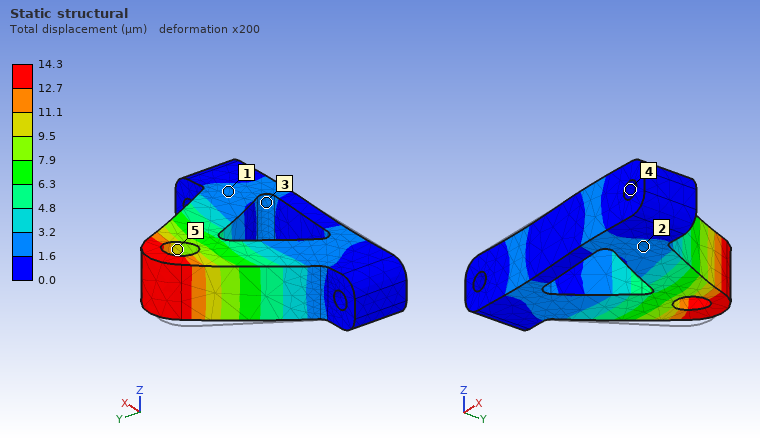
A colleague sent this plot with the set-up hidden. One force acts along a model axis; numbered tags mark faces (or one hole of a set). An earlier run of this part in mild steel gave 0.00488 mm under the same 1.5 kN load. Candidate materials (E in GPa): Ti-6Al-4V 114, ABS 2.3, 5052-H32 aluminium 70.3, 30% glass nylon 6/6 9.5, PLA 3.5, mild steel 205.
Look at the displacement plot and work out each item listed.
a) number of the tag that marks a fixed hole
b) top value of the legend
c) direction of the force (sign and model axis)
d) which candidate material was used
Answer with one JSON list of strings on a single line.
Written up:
["4", "14.3 µm", "+X", "5052-H32 aluminium"]
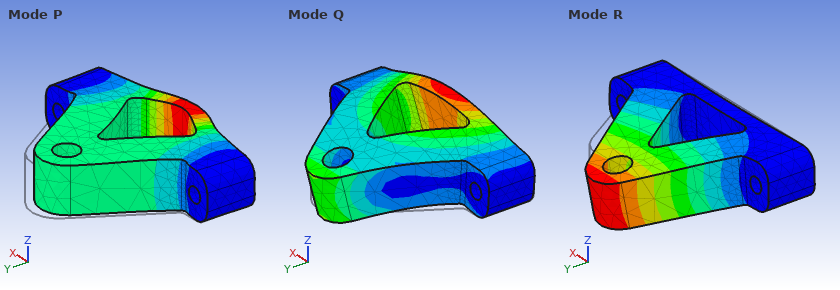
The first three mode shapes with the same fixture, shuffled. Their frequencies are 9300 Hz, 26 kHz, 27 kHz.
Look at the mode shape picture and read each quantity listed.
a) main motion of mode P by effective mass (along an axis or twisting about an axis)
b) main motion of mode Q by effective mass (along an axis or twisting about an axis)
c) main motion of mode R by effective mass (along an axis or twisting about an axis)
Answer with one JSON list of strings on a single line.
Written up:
["along Y", "along Z", "along Z"]
